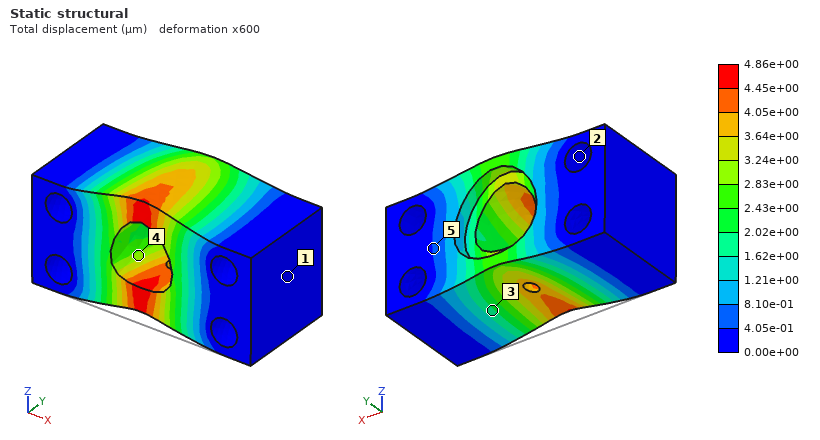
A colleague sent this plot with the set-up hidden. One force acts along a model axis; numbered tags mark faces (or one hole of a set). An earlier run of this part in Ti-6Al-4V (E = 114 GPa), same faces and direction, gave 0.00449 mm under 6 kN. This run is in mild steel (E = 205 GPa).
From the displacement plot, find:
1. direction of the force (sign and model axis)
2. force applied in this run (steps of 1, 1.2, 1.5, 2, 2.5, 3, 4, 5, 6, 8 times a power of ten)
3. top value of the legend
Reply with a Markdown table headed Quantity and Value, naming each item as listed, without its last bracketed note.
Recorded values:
| Quantity | Value |
|---|---|
| direction of the force | +Z |
| force applied in this run | 12 kN |
| top value of the legend | 4.86e+00 µm |
